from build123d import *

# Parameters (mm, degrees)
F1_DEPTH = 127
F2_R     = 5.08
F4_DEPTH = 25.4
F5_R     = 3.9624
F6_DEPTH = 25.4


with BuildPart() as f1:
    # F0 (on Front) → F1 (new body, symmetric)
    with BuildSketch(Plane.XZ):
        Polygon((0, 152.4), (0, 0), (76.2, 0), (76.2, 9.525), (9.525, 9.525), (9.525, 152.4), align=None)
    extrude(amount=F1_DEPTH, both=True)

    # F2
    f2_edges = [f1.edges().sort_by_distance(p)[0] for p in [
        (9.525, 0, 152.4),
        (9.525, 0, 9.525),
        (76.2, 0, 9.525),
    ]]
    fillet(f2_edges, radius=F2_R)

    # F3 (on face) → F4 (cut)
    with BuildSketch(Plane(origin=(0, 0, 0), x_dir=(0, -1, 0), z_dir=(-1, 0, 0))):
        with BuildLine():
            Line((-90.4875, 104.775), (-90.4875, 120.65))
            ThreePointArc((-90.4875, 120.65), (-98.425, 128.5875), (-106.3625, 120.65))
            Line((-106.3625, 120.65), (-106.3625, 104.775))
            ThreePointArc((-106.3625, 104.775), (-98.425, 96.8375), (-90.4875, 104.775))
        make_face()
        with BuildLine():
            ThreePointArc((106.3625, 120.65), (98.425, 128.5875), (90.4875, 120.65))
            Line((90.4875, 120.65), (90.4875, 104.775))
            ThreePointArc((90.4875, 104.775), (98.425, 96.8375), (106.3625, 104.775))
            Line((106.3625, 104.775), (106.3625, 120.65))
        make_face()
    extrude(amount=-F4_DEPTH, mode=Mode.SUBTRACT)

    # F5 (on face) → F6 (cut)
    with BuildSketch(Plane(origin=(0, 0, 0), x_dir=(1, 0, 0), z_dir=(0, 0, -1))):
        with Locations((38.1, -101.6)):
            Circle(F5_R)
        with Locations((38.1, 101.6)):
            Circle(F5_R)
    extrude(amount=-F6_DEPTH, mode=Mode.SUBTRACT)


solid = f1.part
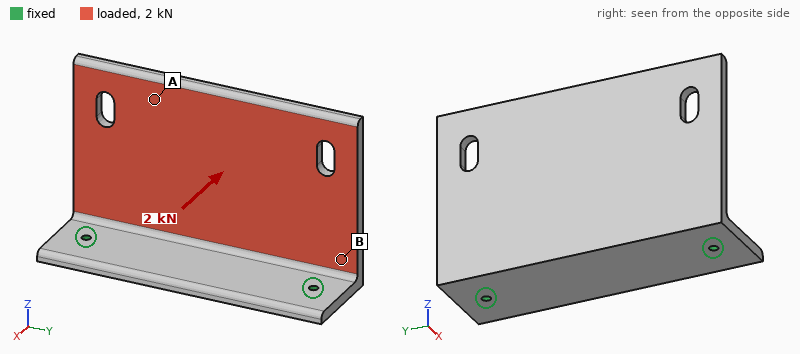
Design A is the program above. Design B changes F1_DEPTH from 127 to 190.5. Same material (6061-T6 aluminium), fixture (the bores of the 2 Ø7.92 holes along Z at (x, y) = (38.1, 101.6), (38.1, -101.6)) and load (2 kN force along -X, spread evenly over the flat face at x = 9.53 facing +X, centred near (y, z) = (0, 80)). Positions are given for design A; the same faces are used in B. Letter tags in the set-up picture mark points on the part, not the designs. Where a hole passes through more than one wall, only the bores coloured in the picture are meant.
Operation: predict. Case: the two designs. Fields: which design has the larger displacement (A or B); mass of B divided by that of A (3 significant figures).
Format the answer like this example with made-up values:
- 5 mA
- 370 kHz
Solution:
- A
- 1.51
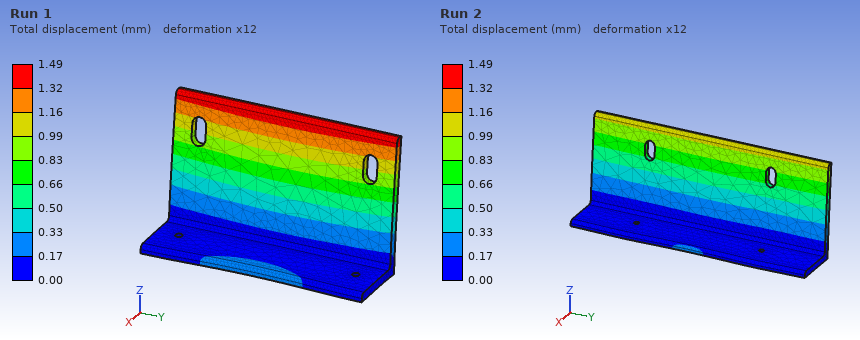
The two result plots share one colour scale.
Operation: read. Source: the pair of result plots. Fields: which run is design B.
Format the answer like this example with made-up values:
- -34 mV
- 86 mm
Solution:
- Run 2
